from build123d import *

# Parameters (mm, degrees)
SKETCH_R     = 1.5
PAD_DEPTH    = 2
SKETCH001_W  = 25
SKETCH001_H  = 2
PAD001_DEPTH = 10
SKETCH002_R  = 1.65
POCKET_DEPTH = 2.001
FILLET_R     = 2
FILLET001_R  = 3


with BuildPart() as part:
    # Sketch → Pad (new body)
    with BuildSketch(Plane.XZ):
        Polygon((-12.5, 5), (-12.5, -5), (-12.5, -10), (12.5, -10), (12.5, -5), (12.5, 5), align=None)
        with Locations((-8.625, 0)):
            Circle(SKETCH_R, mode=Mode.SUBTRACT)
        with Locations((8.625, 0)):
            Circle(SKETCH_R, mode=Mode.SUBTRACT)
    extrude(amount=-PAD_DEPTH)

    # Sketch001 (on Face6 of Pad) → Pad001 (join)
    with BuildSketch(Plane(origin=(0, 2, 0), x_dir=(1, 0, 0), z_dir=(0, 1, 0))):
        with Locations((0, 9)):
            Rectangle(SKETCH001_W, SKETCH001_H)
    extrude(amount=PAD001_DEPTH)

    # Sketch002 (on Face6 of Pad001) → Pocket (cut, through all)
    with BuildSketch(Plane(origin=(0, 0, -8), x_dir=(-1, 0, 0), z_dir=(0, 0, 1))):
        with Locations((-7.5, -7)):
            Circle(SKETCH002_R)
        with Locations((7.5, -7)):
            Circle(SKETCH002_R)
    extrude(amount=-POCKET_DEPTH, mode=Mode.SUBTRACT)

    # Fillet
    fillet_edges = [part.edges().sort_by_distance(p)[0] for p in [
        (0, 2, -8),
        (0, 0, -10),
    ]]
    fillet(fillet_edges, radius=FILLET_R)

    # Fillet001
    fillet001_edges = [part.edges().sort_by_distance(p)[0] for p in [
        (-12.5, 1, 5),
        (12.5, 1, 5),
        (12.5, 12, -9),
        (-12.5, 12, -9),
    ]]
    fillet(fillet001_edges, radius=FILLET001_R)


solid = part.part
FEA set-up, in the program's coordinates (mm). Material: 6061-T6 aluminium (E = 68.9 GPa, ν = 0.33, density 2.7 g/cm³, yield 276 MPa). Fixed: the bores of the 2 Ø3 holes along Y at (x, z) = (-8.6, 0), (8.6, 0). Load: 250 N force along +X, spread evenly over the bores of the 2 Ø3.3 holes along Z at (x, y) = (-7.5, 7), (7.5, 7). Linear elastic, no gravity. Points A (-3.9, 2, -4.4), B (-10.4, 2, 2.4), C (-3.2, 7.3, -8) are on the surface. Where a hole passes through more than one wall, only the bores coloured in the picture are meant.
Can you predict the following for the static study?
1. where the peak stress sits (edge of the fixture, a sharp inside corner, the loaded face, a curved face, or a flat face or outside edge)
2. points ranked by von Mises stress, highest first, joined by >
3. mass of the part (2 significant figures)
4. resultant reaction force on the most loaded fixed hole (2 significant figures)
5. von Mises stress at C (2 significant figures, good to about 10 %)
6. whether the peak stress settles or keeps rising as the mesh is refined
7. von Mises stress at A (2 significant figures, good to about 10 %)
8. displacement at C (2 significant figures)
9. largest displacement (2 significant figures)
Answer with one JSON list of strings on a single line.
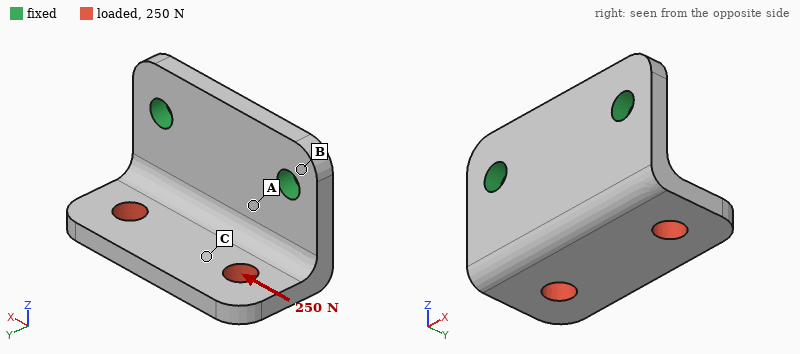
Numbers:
["edge of the fixture", "A > C > B", "3.2 g", "190 N", "18 MPa", "keeps rising", "32 MPa", "15 µm", "32 µm"]
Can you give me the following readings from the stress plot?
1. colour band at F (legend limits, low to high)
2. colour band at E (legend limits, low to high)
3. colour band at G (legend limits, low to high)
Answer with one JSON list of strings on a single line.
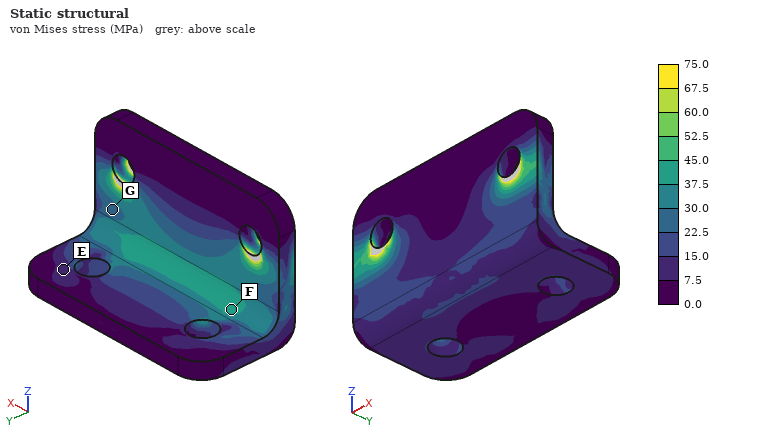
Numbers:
["37.5 to 45.0 MPa", "7.5 to 15.0 MPa", "22.5 to 30.0 MPa"]
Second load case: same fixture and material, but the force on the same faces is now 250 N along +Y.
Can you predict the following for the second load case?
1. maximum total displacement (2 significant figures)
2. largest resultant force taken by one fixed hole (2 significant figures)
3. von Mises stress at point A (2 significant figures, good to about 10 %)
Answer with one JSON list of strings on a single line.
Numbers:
["0.10 mm", "130 N", "54 MPa"]
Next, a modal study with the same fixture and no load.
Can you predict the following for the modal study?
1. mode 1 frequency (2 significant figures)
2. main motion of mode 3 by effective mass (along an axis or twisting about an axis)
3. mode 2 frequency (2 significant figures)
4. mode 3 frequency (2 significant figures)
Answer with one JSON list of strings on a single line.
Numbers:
["6200 Hz", "along Y", "11 kHz", "18 kHz"]
